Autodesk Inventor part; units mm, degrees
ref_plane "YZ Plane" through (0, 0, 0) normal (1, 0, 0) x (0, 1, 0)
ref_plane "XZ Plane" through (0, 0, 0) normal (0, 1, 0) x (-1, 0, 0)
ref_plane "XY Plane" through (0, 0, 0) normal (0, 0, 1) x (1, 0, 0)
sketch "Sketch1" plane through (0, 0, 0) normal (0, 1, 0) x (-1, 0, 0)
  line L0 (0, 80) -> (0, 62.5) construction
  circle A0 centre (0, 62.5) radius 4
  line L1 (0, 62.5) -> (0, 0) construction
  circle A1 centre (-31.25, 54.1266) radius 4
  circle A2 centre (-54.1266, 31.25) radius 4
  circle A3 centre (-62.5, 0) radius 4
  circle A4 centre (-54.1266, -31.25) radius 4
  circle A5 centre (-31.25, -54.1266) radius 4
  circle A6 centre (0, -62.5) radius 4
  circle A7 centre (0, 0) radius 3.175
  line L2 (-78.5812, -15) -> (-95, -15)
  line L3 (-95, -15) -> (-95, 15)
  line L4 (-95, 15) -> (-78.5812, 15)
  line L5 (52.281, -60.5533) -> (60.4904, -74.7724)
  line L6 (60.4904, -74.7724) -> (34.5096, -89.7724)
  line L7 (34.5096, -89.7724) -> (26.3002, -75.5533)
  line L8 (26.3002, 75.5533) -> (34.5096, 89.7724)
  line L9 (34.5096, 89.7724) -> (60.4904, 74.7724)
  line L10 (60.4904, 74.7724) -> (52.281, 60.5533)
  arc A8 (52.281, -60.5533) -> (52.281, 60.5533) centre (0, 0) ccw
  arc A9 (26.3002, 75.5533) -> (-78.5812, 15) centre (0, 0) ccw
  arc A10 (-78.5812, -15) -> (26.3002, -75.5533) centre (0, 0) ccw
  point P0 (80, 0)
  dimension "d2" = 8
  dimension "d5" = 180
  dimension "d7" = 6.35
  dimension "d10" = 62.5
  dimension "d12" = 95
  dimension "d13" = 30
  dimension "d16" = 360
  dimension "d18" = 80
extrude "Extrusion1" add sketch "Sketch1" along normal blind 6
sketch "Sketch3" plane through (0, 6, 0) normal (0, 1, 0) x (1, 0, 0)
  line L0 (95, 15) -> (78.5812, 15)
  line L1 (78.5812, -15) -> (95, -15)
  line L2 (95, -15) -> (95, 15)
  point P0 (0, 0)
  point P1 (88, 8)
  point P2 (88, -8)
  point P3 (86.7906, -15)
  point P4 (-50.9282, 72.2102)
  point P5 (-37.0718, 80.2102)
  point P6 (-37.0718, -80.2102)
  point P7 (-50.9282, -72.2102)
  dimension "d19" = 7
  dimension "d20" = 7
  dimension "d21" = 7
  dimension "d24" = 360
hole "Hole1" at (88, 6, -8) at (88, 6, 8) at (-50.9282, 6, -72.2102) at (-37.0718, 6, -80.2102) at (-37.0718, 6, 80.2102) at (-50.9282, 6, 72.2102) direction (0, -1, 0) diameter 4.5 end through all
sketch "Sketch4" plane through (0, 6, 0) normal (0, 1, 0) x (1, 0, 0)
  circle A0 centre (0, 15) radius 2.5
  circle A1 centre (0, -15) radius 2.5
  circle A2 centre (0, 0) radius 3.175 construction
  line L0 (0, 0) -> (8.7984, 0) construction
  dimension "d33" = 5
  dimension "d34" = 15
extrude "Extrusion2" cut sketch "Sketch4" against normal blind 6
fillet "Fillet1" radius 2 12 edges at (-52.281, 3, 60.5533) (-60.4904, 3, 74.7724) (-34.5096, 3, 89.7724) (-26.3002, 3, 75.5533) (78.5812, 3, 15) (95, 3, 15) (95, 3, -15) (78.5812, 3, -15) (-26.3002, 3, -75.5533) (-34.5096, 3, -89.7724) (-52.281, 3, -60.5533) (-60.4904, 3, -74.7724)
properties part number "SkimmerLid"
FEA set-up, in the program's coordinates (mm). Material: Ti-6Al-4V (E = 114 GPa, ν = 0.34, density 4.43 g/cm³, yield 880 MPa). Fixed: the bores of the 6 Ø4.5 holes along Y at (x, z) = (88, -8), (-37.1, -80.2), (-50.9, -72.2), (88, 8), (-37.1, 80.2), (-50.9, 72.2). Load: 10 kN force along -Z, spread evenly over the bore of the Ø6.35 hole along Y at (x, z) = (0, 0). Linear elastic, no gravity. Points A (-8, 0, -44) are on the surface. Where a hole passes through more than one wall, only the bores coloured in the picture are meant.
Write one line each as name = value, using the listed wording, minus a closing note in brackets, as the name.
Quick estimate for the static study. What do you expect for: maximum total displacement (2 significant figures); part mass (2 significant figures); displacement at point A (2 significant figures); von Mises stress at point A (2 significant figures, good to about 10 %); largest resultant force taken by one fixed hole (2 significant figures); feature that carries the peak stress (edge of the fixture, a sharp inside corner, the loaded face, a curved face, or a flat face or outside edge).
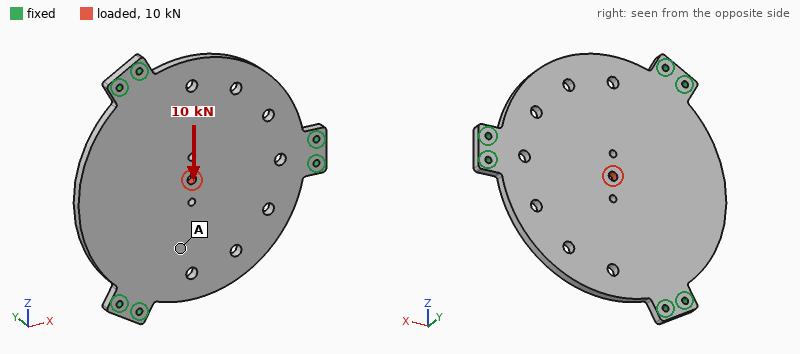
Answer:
maximum total displacement = 22 µm
part mass = 560 g
displacement at point A = 10 µm
von Mises stress at point A = 15 MPa
largest resultant force taken by one fixed hole = 2.6 kN
feature that carries the peak stress = the loaded face
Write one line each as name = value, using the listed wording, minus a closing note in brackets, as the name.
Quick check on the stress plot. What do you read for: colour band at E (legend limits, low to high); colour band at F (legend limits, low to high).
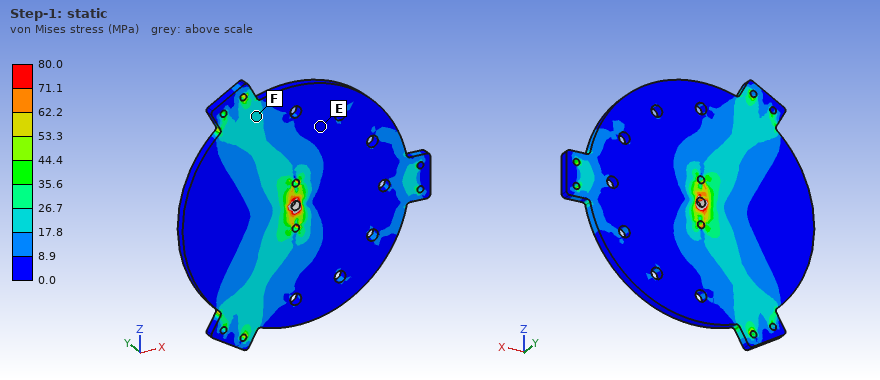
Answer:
colour band at E = 0.0 to 8.9 MPa
colour band at F = 17.8 to 26.7 MPa
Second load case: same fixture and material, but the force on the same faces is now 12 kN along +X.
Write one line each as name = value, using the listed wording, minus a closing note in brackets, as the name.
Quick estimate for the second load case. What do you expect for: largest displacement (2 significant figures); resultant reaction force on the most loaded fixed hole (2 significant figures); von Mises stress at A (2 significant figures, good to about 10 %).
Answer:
largest displacement = 26 µm
resultant reaction force on the most loaded fixed hole = 2.8 kN
von Mises stress at A = 10 MPa
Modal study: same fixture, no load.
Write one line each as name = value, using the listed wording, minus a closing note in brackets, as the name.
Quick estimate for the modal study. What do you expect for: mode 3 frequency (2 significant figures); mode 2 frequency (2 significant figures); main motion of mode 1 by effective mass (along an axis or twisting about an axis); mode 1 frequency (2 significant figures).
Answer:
mode 3 frequency = 1300 Hz
mode 2 frequency = 1300 Hz
main motion of mode 1 by effective mass = along Y
mode 1 frequency = 1100 Hz
